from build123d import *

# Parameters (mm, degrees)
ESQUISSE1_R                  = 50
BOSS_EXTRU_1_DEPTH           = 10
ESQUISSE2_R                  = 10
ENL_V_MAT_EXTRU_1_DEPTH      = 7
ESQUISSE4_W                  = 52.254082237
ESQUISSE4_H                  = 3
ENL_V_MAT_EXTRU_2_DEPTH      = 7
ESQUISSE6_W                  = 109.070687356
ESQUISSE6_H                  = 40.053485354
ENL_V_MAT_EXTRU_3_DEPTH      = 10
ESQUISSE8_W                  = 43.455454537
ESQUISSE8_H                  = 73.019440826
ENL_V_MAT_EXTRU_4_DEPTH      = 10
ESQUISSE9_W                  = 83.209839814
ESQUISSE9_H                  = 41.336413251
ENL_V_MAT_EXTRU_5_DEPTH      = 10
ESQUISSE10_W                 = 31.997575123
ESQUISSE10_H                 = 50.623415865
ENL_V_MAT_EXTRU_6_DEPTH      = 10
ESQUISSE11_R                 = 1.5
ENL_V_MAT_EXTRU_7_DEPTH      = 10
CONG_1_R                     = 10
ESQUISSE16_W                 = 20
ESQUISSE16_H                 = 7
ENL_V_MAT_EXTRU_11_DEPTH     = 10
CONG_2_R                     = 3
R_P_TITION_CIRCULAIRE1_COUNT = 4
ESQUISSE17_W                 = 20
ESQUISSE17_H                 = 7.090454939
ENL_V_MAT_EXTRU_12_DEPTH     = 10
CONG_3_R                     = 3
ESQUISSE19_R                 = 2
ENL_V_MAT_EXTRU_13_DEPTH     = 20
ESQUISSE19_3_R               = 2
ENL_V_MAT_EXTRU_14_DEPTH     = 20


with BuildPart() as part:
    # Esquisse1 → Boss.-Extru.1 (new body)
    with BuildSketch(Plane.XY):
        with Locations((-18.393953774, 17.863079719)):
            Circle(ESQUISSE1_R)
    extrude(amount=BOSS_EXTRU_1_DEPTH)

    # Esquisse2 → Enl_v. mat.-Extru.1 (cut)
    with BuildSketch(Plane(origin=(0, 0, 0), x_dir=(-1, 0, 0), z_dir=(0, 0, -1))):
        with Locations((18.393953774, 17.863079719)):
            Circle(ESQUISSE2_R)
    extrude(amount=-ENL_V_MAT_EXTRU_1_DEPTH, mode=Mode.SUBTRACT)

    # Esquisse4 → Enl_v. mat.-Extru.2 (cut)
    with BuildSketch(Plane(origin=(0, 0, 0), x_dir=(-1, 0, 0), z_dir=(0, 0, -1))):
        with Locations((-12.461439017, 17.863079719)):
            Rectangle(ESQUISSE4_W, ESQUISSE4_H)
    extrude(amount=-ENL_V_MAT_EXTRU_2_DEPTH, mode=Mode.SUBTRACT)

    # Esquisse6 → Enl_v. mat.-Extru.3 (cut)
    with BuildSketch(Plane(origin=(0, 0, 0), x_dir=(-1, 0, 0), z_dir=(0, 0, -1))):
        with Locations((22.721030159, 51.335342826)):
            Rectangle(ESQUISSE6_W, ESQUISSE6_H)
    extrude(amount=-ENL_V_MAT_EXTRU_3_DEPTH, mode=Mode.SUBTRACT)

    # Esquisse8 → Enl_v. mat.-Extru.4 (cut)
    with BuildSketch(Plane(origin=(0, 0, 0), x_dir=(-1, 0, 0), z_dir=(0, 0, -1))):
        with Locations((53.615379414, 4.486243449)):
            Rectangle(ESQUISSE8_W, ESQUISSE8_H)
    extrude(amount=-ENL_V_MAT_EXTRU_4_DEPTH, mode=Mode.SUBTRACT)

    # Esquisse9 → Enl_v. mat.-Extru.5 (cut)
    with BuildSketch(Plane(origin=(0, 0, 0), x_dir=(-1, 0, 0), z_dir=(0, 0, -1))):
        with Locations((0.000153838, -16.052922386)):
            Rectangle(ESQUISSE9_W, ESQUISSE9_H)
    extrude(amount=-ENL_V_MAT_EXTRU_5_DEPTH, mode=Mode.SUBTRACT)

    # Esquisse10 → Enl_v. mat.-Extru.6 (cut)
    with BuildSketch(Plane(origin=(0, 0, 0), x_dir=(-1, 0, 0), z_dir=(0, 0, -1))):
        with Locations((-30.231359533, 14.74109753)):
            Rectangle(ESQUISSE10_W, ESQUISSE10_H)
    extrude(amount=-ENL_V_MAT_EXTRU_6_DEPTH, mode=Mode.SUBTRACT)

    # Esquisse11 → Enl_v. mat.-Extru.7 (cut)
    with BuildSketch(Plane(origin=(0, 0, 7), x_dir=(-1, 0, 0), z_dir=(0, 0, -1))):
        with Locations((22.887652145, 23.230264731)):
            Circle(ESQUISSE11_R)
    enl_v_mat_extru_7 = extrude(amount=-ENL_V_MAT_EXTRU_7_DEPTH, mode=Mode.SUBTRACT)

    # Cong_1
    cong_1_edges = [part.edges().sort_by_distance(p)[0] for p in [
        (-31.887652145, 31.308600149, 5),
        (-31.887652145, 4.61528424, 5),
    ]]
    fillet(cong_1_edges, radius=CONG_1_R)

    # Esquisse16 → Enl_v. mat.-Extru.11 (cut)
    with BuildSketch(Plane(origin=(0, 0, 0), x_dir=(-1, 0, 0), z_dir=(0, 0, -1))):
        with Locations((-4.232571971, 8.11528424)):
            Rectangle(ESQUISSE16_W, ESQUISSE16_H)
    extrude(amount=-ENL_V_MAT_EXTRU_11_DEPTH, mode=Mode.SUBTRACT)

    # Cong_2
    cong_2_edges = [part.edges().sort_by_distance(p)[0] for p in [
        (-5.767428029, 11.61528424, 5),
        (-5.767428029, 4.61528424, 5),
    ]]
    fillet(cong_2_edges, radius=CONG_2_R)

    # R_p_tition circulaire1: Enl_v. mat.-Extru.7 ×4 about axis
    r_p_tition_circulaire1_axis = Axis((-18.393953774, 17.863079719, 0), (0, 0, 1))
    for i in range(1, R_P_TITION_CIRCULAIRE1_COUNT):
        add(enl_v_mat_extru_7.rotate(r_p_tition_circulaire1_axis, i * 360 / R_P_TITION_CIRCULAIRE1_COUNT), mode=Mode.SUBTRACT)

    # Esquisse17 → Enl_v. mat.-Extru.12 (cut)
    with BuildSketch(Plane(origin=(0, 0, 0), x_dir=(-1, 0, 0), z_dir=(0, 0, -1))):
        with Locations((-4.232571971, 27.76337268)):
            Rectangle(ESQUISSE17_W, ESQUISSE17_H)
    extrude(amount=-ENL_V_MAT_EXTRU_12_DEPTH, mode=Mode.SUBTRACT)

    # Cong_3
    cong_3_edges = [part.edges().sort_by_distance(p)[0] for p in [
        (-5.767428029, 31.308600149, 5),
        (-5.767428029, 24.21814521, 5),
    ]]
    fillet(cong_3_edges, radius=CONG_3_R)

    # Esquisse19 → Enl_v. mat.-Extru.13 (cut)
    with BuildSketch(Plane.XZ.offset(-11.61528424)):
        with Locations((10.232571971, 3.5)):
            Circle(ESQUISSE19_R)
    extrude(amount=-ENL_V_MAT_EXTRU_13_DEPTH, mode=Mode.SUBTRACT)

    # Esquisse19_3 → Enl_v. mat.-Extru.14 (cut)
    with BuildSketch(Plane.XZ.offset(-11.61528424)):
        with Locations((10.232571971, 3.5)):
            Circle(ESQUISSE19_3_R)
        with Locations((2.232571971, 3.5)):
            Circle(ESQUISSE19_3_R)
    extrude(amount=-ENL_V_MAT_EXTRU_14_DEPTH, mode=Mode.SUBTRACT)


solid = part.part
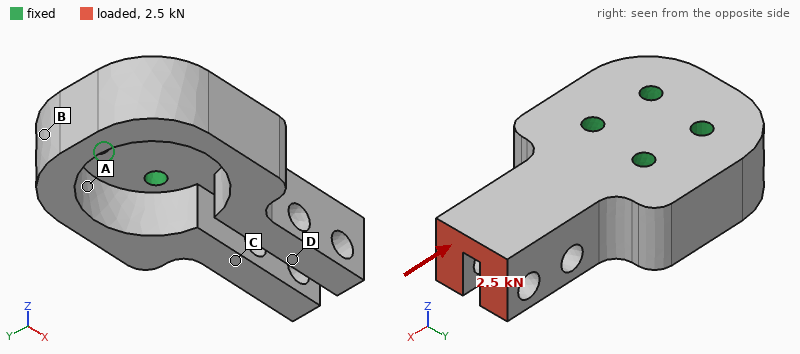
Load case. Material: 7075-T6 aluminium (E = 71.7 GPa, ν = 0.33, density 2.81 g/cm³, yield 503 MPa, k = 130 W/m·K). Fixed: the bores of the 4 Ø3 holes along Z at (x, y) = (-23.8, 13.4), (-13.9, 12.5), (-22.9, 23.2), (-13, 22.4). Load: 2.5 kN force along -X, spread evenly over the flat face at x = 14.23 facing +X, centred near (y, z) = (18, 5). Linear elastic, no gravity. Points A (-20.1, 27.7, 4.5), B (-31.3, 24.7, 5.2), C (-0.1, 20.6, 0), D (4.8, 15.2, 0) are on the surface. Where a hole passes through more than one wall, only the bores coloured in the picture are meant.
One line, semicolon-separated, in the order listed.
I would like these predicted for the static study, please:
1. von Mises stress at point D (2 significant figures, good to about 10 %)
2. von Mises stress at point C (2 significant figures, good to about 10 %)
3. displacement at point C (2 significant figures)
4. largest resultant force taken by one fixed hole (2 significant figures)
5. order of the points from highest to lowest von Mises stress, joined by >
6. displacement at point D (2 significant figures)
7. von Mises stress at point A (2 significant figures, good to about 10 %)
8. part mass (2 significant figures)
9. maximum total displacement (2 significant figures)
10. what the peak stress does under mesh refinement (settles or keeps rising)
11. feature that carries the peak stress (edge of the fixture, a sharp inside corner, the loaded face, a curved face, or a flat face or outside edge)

57 MPa; 38 MPa; 33 µm; 1.1 kN; D > C > A > B; 43 µm; 25 MPa; 17 g; 66 µm; keeps rising; edge of the fixture
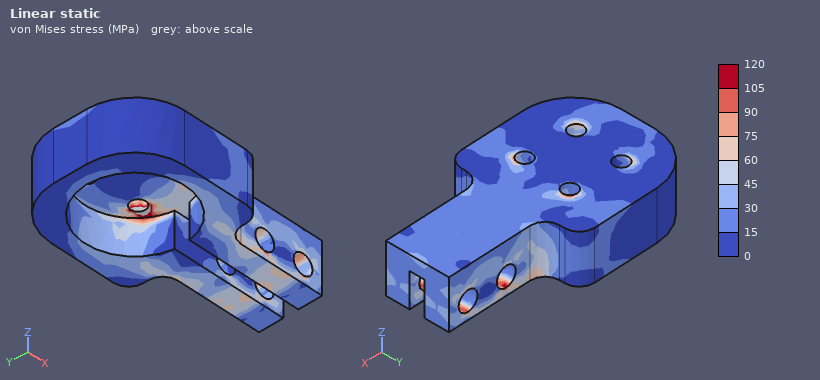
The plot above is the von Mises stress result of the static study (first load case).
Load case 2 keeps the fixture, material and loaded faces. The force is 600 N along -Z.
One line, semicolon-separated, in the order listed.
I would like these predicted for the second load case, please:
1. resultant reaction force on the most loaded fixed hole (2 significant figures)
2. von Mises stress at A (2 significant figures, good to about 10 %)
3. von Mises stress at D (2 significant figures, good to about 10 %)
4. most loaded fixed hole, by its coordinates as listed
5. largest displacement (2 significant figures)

940 N; 44 MPa; 36 MPa; (-13, 22.4); 0.17 mm
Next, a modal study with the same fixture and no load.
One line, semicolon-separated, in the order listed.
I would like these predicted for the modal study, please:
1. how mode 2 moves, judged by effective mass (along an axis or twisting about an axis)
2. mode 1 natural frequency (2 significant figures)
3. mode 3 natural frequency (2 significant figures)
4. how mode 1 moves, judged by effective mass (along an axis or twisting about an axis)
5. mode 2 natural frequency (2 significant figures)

along Y; 6700 Hz; 15 kHz; along Z; 12 kHz
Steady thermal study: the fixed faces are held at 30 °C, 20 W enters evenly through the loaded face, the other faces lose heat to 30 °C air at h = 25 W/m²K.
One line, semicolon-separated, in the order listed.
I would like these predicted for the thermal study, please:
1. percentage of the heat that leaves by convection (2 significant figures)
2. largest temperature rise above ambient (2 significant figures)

5.9 %; 49 K
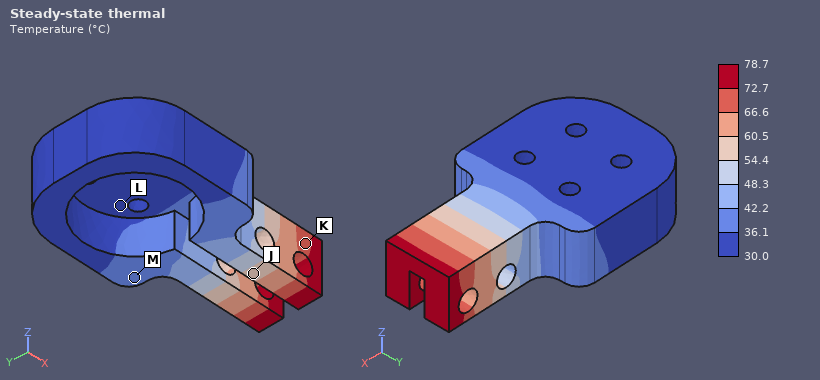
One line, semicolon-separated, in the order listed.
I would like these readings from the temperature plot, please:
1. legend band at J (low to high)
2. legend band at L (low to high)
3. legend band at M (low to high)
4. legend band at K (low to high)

54.4 to 60.5 °C; 30.0 to 36.1 °C; 36.1 to 42.2 °C; 66.6 to 72.7 °C
